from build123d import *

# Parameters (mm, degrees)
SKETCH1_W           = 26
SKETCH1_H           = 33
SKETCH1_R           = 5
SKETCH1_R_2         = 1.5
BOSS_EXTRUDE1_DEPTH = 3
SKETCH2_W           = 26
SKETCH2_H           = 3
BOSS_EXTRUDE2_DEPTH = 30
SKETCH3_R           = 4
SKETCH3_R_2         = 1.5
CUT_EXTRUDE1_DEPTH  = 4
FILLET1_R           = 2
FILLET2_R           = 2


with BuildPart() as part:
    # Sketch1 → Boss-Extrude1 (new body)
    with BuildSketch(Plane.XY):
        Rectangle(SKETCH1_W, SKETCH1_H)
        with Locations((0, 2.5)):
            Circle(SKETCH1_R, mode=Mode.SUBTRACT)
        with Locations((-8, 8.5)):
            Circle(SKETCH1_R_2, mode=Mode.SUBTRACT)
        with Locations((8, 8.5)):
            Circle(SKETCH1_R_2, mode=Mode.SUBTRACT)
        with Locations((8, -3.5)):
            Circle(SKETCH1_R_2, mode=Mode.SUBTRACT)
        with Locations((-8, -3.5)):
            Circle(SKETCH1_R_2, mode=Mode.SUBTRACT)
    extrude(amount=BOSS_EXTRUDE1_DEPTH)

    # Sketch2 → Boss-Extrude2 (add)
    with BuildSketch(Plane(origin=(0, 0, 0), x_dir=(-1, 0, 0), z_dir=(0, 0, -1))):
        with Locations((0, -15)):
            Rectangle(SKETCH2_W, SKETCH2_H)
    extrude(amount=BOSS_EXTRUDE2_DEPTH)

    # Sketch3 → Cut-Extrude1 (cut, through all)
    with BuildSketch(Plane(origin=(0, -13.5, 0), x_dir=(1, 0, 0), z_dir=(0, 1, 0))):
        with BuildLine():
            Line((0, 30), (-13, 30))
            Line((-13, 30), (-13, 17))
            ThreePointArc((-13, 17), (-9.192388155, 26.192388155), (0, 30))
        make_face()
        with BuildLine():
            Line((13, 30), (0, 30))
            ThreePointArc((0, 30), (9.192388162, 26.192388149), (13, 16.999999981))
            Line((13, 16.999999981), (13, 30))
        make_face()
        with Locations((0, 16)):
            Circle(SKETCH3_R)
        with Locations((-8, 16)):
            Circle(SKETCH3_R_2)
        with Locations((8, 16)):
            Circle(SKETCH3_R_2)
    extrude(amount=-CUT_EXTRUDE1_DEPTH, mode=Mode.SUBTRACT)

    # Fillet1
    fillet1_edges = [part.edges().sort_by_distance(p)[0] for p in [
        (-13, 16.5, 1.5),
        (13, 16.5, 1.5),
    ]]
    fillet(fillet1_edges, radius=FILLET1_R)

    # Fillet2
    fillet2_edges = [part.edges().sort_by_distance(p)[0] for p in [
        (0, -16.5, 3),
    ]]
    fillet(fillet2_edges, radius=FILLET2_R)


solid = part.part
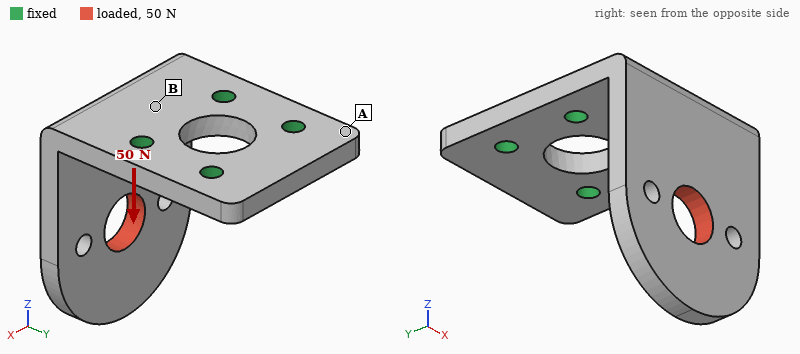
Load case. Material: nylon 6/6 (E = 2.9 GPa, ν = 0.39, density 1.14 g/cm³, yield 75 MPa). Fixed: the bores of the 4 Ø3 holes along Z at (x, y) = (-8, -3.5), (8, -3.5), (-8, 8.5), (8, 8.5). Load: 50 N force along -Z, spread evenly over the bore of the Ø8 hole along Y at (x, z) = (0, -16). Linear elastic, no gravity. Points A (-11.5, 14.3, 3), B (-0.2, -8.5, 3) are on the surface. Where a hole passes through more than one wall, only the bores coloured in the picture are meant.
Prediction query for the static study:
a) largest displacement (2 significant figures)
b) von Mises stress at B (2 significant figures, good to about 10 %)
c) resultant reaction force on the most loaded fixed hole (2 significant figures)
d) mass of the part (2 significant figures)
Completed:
0.61 mm
5.6 MPa
28 N
4.7 g
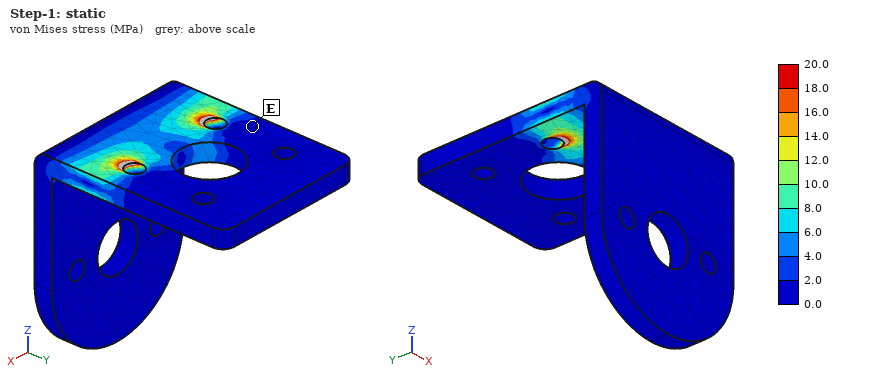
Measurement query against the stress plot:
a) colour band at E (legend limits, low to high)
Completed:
0.0 to 2.0 MPa
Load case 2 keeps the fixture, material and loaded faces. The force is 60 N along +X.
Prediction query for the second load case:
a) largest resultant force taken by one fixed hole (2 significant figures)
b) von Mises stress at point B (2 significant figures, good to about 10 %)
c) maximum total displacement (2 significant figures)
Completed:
75 N
6.8 MPa
0.59 mm
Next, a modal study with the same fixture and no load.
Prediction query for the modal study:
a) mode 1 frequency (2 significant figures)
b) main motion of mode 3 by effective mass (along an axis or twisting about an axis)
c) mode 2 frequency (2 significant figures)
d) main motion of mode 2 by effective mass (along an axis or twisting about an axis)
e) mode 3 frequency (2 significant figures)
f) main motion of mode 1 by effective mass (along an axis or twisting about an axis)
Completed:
610 Hz
along Z
1300 Hz
along X
2300 Hz
along Y
